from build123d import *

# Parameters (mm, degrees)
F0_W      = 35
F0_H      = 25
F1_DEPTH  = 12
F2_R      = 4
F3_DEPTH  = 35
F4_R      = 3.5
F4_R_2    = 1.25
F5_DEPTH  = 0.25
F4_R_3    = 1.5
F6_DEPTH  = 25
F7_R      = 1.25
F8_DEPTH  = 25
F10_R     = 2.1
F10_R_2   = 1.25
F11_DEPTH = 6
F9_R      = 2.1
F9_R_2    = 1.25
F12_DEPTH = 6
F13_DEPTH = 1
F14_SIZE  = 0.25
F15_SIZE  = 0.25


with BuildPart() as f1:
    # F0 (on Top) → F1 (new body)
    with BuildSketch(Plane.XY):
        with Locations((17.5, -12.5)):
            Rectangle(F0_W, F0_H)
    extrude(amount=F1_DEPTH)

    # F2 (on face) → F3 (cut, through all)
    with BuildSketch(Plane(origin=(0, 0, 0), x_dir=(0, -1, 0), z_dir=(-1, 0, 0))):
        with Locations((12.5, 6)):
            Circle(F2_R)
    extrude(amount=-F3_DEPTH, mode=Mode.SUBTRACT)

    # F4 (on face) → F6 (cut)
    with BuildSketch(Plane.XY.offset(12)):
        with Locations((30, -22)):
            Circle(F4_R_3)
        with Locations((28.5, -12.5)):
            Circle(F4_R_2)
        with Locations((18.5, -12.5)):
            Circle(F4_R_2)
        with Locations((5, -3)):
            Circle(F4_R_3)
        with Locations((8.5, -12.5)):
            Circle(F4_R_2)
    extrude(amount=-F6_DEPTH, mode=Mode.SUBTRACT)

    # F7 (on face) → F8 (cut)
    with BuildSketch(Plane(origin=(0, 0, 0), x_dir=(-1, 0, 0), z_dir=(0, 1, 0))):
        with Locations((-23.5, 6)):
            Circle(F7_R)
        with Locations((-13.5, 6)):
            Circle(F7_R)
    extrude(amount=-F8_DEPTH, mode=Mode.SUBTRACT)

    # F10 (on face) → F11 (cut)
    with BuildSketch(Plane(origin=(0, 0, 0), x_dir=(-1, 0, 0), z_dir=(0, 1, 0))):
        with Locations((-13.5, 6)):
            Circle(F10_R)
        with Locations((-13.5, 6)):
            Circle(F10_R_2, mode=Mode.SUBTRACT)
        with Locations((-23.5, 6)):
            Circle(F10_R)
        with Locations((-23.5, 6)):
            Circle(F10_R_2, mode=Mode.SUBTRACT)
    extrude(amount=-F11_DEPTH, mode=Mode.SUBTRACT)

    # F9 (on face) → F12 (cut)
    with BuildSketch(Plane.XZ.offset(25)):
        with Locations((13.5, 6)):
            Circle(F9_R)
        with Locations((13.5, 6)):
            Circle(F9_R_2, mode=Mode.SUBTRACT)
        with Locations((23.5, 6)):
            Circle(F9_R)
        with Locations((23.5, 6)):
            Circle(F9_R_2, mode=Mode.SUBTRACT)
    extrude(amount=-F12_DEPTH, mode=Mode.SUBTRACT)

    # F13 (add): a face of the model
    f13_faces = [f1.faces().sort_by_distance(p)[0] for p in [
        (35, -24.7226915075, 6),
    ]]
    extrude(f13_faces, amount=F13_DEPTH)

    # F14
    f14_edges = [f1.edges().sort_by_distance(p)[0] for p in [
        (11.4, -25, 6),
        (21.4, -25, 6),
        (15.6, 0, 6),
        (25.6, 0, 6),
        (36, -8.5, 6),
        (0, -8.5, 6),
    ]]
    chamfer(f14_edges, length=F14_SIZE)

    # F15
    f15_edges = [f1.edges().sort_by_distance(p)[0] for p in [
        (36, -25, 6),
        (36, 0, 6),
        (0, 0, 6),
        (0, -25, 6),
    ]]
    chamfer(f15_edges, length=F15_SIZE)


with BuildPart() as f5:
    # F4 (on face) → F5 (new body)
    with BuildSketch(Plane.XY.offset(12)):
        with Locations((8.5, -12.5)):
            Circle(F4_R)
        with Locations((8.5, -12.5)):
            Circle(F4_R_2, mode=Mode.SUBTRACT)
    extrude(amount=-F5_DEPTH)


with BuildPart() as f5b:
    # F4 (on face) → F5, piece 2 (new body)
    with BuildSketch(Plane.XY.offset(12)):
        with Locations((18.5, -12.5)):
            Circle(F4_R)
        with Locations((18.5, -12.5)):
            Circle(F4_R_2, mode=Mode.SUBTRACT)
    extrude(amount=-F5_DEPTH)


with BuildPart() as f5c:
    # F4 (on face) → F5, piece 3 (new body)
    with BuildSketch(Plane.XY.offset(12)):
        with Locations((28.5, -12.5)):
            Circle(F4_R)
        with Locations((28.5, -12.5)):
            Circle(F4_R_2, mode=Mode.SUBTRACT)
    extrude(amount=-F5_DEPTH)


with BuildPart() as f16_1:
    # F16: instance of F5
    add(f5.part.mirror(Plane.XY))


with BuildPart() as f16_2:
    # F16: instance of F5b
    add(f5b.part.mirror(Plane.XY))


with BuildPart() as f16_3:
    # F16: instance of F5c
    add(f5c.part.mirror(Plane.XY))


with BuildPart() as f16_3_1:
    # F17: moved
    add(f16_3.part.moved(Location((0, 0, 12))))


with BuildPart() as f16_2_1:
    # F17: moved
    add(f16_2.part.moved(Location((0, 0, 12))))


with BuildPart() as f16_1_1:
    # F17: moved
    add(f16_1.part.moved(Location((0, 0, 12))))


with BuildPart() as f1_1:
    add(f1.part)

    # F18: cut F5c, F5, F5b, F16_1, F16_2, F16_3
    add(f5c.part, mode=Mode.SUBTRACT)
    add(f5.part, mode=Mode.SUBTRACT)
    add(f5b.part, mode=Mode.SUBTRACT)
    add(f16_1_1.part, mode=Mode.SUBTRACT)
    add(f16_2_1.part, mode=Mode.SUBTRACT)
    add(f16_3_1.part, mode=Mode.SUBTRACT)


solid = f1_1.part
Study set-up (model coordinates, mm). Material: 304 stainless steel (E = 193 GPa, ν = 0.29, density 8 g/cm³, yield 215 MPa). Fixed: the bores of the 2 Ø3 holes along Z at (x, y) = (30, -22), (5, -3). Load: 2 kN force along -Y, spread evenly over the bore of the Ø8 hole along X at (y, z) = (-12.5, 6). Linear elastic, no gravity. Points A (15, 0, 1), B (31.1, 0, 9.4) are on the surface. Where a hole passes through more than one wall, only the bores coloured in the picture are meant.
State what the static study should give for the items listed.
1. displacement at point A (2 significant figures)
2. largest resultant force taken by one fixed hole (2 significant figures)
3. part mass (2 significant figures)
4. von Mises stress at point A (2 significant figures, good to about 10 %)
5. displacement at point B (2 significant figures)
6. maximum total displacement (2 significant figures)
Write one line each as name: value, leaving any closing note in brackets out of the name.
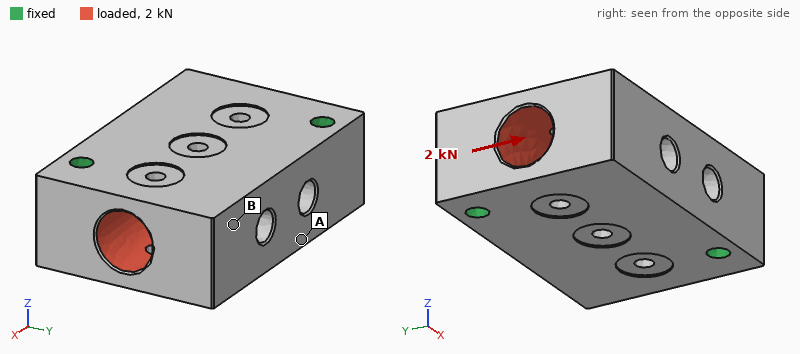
displacement at point A: 0.77 µm
largest resultant force taken by one fixed hole: 1.0 kN
part mass: 67 g
von Mises stress at point A: 5.5 MPa
displacement at point B: 0.87 µm
maximum total displacement: 1.0 µm
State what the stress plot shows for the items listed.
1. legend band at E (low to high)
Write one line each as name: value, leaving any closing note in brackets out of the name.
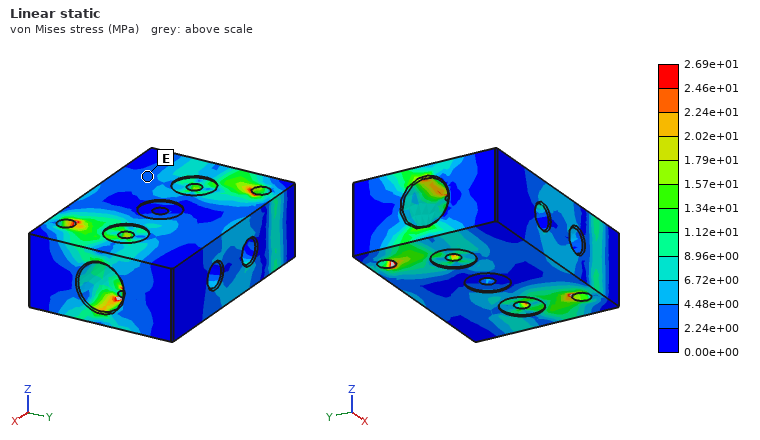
legend band at E: 2.24e+00 to 4.48e+00 MPa
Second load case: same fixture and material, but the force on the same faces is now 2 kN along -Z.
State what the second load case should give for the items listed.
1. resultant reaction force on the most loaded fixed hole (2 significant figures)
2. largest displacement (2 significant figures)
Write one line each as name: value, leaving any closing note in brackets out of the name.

resultant reaction force on the most loaded fixed hole: 1.0 kN
largest displacement: 3.5 µm
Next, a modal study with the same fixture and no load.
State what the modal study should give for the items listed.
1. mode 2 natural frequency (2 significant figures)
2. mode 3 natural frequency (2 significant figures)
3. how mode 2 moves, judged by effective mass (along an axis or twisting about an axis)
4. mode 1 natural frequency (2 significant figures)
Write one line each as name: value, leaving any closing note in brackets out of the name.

mode 2 natural frequency: 17 kHz
mode 3 natural frequency: 29 kHz
how mode 2 moves, judged by effective mass: along Z
mode 1 natural frequency: 14 kHz
